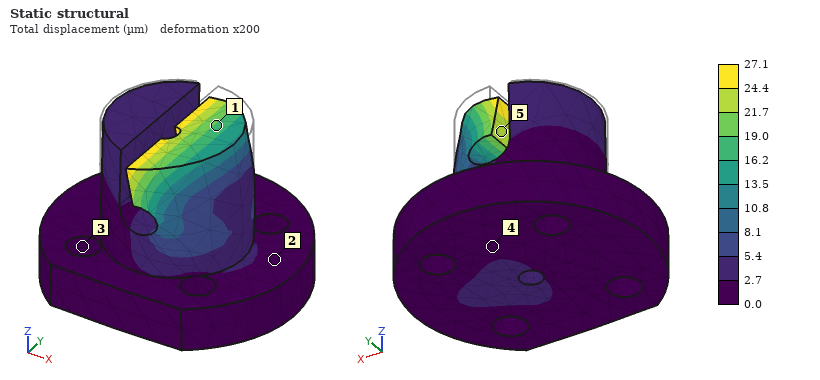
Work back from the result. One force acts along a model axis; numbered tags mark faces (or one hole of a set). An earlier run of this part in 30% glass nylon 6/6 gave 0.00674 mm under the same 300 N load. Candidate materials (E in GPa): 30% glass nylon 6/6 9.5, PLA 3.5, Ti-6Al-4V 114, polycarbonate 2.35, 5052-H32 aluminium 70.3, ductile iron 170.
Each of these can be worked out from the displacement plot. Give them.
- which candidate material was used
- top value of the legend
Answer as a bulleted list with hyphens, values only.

- polycarbonate
- 27.1 µm
